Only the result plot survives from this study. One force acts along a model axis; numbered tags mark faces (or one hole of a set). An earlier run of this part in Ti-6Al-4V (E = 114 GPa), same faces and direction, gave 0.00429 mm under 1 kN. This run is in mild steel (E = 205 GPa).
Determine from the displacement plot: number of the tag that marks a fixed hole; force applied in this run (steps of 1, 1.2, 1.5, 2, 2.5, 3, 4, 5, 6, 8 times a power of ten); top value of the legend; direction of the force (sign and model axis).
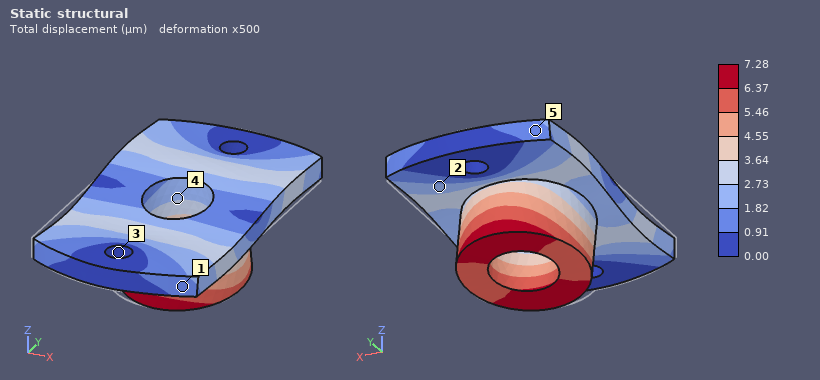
3
3 kN
7.28 µm
+Y
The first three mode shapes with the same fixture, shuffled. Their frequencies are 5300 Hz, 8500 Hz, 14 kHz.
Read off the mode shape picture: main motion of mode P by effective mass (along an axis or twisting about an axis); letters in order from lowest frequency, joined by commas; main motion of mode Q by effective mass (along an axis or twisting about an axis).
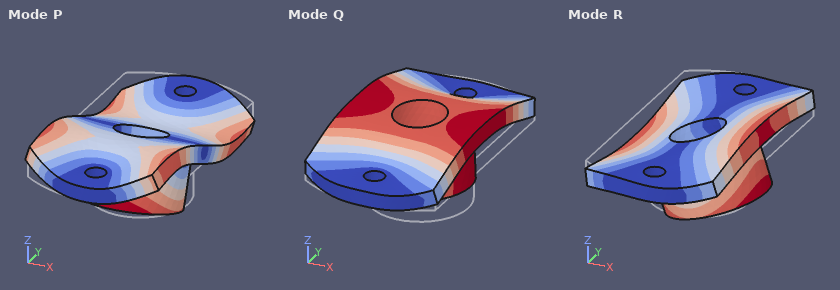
along Y
R, Q, P
along Z
